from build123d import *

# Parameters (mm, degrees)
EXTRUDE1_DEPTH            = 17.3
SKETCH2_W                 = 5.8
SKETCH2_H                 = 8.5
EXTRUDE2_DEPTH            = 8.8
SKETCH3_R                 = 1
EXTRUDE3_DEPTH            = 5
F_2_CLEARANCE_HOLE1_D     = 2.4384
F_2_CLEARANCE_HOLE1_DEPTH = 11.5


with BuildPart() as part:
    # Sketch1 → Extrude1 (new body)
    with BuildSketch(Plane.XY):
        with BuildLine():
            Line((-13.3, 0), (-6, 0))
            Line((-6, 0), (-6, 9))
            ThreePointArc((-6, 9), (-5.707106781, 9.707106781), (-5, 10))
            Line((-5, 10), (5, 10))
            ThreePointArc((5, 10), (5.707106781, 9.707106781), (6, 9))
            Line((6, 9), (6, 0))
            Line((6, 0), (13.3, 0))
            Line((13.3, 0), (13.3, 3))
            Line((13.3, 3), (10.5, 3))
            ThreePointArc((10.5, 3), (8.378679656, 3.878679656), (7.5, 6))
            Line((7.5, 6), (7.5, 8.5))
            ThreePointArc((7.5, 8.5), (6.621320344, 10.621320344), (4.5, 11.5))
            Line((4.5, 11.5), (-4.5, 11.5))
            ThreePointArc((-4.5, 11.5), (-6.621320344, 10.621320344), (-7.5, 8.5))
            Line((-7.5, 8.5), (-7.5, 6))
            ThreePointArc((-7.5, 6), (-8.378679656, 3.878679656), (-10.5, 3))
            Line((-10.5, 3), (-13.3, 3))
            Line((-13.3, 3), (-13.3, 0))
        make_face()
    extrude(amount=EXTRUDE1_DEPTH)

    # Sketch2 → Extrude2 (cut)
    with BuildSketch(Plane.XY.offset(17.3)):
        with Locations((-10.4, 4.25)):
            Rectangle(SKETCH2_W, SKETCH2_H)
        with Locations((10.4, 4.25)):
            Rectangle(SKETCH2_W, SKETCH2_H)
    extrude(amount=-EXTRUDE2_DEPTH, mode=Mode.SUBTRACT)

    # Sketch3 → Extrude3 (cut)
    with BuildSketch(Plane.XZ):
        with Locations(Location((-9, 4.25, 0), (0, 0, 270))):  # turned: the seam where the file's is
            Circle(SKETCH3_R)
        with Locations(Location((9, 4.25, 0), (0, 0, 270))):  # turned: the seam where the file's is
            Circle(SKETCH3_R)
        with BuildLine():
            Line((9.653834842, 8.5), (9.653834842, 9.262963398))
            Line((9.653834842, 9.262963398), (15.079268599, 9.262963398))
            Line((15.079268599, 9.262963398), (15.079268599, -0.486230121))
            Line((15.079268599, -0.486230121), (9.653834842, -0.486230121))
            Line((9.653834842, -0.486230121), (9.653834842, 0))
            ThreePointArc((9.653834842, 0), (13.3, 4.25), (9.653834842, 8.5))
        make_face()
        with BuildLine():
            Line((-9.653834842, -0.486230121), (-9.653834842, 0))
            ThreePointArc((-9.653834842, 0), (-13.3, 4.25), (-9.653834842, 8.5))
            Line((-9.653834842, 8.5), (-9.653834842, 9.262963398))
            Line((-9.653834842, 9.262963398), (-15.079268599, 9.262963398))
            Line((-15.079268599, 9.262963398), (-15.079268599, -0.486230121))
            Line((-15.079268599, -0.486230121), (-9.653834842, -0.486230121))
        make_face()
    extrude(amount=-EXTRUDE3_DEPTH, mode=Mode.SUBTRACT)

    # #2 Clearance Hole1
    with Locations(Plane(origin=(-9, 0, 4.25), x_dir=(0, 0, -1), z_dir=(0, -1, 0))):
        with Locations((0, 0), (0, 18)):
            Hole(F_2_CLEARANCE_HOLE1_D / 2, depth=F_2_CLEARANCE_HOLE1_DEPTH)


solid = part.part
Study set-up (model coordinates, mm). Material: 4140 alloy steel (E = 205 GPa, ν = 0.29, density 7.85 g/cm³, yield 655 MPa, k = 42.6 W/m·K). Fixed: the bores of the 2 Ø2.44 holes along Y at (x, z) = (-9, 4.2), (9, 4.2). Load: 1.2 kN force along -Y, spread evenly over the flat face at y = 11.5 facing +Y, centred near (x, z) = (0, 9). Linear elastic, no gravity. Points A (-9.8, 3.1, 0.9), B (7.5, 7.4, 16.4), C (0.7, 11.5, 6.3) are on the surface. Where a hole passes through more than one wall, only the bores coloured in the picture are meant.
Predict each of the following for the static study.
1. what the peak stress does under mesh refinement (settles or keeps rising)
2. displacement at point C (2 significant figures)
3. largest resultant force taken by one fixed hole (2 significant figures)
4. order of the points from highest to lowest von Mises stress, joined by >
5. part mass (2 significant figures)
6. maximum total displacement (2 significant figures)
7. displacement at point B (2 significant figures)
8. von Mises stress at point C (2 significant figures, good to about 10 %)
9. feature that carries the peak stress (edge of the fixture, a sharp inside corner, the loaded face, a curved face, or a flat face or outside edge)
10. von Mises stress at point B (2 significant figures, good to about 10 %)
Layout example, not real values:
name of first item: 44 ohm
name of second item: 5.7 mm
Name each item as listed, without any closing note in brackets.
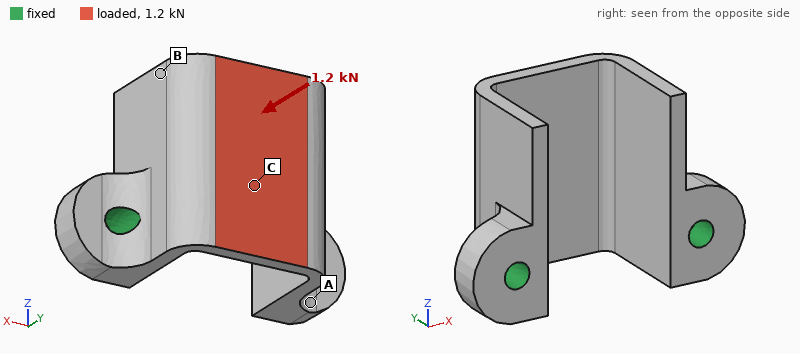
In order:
what the peak stress does under mesh refinement: keeps rising
displacement at point C: 20 µm
largest resultant force taken by one fixed hole: 660 N
order of the points from highest to lowest von Mises stress, joined by >: C > B > A
part mass: 8.6 g
maximum total displacement: 38 µm
displacement at point B: 14 µm
von Mises stress at point C: 180 MPa
feature that carries the peak stress: edge of the fixture
von Mises stress at point B: 85 MPa
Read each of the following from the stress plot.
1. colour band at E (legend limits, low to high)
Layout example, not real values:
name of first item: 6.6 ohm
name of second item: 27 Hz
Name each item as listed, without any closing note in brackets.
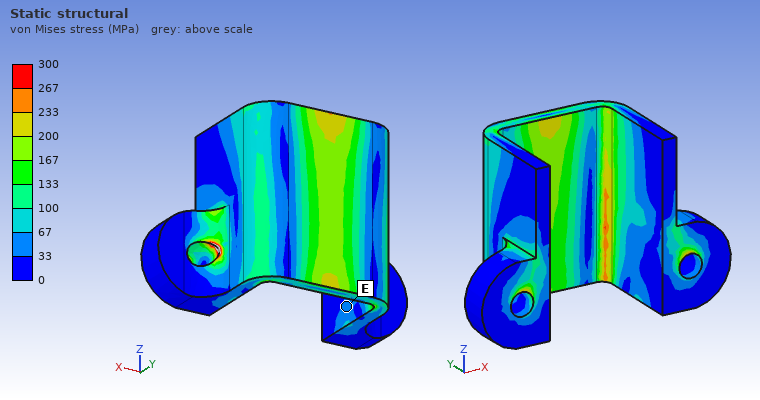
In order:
colour band at E: 33 to 67 MPa
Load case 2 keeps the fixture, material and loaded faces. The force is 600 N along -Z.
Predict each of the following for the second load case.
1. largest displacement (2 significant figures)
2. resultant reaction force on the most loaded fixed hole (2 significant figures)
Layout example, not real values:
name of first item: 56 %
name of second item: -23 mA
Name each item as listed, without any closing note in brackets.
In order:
largest displacement: 17 µm
resultant reaction force on the most loaded fixed hole: 300 N
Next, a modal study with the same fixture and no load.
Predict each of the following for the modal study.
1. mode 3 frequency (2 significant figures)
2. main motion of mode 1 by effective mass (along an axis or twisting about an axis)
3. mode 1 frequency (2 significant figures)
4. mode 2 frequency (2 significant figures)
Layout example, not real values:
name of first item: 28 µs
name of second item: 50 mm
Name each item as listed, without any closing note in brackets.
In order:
mode 3 frequency: 19 kHz
main motion of mode 1 by effective mass: along X
mode 1 frequency: 13 kHz
mode 2 frequency: 17 kHz
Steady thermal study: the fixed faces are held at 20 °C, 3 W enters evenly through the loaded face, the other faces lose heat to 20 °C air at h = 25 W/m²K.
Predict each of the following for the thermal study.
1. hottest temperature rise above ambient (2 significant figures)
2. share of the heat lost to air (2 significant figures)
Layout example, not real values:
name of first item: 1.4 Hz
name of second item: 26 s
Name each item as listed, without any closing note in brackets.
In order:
hottest temperature rise above ambient: 20 K
share of the heat lost to air: 9.4 %
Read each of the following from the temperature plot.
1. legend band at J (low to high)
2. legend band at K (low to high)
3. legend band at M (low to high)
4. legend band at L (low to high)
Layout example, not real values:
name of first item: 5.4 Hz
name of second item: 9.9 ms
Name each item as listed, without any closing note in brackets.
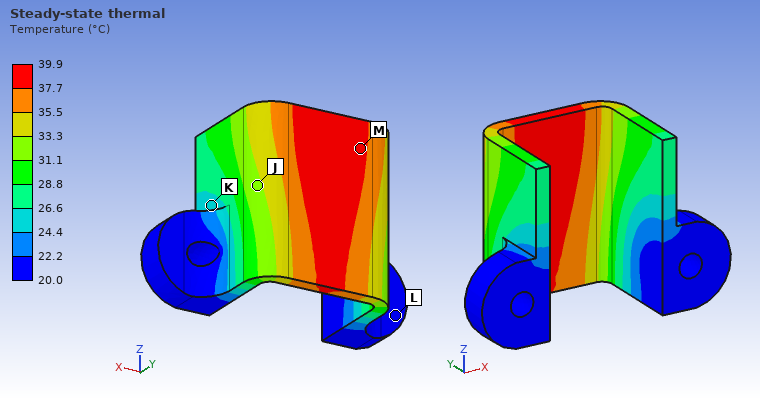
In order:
legend band at J: 31.1 to 33.3 °C
legend band at K: 24.4 to 26.6 °C
legend band at M: 37.7 to 39.9 °C
legend band at L: 20.0 to 22.2 °C
